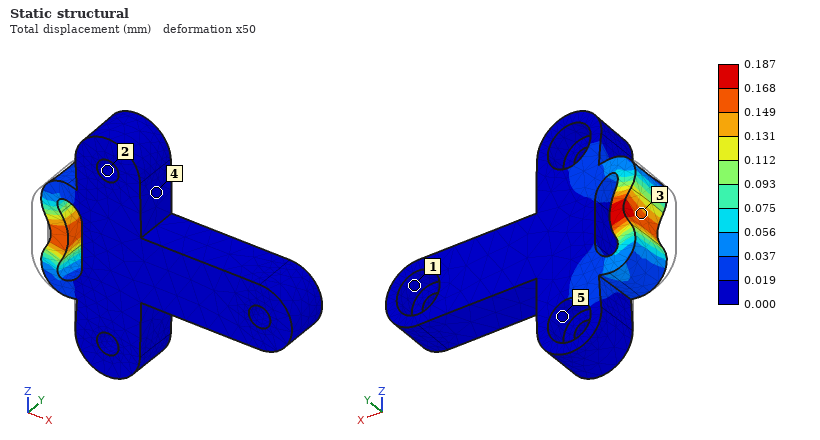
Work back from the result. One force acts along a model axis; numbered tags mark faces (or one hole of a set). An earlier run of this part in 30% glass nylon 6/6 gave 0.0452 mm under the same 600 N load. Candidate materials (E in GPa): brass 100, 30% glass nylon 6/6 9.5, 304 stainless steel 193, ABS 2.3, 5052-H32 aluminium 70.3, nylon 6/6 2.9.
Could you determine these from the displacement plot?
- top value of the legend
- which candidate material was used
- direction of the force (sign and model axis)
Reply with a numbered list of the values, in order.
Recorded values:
1. 0.187 mm
2. ABS
3. +X
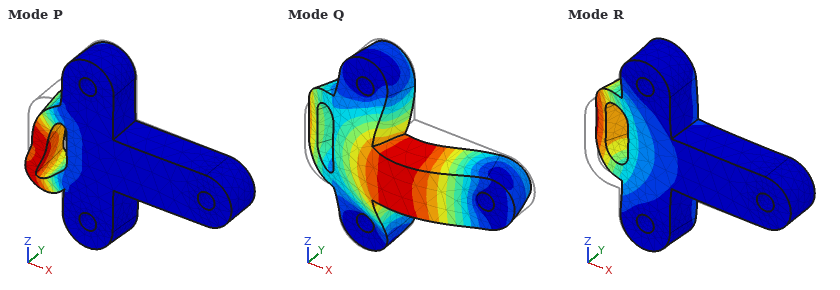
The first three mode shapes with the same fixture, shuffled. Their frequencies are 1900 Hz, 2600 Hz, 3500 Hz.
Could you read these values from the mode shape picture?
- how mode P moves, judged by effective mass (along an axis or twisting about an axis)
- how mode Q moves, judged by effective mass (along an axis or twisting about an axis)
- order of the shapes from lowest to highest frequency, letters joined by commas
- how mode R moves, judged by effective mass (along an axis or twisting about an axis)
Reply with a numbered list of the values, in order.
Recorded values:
1. along Z
2. along Y
3. R, Q, P
4. along Y
